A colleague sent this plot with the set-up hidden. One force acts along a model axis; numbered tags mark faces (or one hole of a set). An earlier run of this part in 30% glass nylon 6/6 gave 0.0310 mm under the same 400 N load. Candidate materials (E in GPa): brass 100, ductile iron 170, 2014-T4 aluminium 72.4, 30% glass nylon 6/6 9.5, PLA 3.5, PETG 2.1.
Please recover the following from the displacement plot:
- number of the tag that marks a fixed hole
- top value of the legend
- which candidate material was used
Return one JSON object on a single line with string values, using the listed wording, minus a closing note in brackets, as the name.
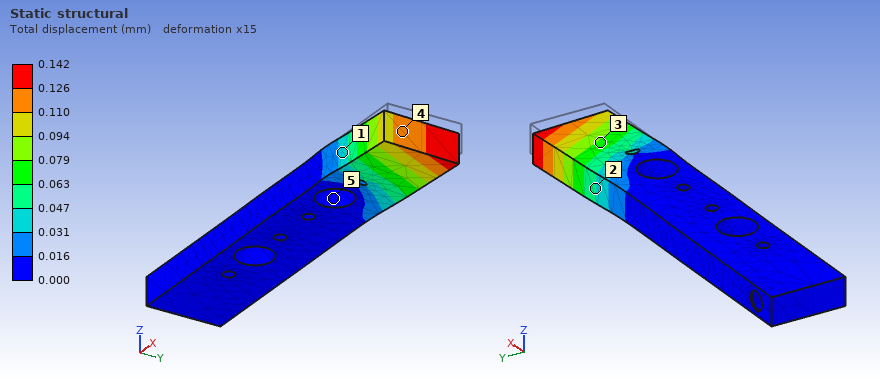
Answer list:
{"number of the tag that marks a fixed hole": "5", "top value of the legend": "0.142 mm", "which candidate material was used": "PETG"}
